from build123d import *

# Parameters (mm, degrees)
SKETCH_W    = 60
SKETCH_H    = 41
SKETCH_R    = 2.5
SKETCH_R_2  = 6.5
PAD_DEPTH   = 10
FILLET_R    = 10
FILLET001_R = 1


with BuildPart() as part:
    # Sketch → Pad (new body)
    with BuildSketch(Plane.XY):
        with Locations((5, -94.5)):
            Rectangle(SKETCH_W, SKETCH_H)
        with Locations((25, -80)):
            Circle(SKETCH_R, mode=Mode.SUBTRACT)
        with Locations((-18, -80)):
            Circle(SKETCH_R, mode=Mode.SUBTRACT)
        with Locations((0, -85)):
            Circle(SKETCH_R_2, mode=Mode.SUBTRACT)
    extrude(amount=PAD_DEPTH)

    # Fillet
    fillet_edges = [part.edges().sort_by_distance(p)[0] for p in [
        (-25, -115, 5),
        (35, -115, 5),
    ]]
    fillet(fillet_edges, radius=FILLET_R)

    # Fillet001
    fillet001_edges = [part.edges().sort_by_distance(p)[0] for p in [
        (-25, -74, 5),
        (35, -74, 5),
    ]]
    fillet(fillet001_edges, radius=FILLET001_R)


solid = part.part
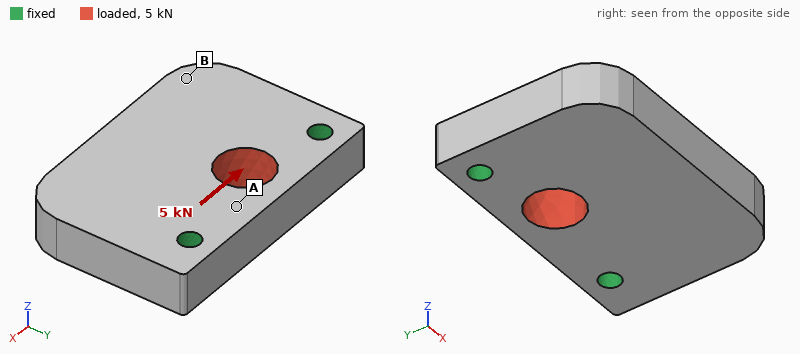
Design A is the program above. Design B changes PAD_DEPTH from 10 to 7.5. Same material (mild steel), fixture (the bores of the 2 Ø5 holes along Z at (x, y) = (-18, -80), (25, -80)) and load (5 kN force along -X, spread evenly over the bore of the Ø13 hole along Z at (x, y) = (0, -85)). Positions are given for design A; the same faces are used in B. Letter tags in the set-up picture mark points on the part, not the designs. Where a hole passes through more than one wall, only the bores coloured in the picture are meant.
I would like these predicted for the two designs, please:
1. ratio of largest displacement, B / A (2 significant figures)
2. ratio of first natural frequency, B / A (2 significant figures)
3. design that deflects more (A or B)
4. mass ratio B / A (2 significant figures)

1.3
0.79
B
0.75
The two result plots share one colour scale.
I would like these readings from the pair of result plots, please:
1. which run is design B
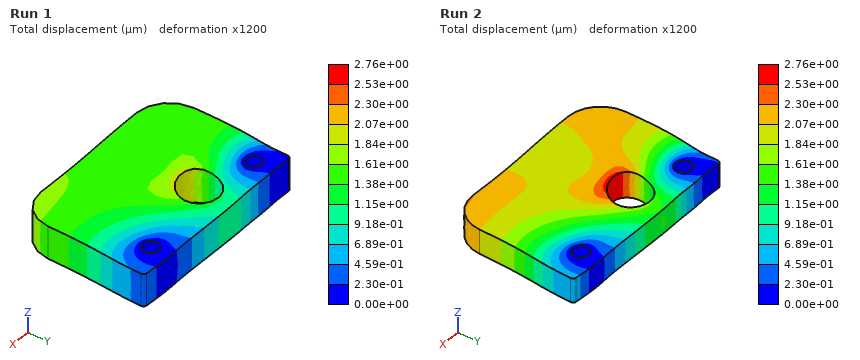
Run 2
